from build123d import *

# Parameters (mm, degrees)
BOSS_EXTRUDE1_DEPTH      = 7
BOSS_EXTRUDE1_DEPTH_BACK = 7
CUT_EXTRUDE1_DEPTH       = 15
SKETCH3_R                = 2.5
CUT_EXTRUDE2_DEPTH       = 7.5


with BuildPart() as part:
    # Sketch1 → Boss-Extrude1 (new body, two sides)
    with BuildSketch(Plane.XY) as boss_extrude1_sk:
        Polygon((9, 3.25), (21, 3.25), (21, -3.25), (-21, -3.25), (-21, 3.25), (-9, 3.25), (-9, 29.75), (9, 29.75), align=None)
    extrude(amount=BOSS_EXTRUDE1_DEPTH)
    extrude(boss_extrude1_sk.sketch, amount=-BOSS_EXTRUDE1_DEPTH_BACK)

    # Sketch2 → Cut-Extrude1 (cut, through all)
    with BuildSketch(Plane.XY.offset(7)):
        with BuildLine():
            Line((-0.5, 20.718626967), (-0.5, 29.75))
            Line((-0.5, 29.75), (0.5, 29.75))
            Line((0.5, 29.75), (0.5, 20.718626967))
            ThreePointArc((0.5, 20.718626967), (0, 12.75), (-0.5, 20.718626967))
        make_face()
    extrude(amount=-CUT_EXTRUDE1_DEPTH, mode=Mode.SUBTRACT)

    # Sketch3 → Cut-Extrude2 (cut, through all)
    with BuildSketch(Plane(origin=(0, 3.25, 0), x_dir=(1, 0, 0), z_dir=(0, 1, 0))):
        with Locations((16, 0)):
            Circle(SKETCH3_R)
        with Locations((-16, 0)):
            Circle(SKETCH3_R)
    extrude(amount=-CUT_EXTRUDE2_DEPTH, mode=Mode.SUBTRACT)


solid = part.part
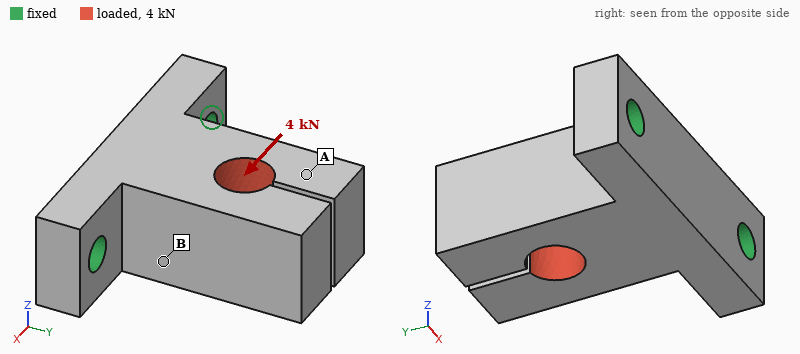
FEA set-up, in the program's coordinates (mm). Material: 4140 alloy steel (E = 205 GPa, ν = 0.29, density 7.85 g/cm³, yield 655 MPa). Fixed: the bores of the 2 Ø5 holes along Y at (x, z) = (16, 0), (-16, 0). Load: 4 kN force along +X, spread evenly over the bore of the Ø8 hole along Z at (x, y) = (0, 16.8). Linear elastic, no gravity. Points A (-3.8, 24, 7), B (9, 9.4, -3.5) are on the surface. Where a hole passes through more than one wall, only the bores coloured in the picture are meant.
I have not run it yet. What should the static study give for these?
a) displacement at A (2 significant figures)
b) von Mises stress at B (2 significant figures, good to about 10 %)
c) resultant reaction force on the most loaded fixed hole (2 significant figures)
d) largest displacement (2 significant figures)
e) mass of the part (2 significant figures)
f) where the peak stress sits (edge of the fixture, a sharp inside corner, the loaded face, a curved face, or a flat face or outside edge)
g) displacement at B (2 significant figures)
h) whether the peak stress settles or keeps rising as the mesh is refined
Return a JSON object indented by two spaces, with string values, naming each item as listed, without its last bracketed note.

{
  "displacement at A": "28 µm",
  "von Mises stress at B": "59 MPa",
  "resultant reaction force on the most loaded fixed hole": "3.4 kN",
  "largest displacement": "38 µm",
  "mass of the part": "74 g",
  "where the peak stress sits": "edge of the fixture",
  "displacement at B": "9.7 µm",
  "whether the peak stress settles or keeps rising as the mesh is refined": "keeps rising"
}
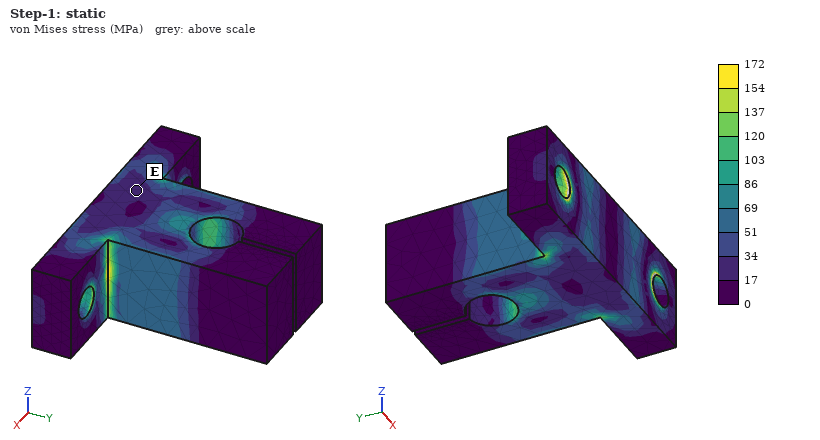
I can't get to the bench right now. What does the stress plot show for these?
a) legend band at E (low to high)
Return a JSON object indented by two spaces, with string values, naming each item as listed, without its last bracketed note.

{
  "legend band at E": "17 to 34 MPa"
}
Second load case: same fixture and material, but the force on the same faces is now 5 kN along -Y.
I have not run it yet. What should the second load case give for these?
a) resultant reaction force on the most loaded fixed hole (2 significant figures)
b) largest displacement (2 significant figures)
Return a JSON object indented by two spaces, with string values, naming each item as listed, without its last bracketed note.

{
  "resultant reaction force on the most loaded fixed hole": "2.7 kN",
  "largest displacement": "22 µm"
}
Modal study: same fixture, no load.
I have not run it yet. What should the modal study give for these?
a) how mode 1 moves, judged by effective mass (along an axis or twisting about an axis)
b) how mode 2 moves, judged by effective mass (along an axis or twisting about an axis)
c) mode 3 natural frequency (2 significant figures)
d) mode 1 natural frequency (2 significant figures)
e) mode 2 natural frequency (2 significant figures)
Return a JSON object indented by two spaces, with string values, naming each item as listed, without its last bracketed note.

{
  "how mode 1 moves, judged by effective mass": "along Z",
  "how mode 2 moves, judged by effective mass": "along X",
  "mode 3 natural frequency": "9400 Hz",
  "mode 1 natural frequency": "5200 Hz",
  "mode 2 natural frequency": "7900 Hz"
}
